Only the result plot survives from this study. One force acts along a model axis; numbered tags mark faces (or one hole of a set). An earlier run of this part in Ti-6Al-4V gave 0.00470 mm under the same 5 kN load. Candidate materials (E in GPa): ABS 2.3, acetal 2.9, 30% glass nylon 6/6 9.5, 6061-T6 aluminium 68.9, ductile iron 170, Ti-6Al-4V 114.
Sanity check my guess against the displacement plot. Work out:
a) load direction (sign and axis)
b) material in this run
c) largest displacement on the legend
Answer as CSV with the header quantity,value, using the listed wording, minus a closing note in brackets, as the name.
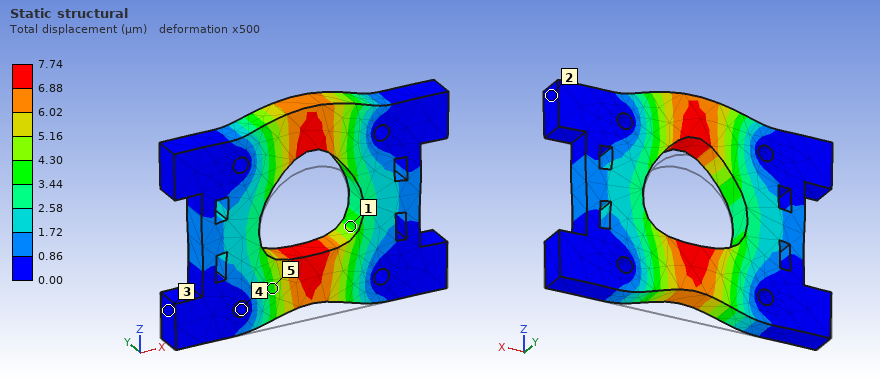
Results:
quantity,value
load direction,+Z
material in this run,6061-T6 aluminium
largest displacement on the legend,7.74 µm
